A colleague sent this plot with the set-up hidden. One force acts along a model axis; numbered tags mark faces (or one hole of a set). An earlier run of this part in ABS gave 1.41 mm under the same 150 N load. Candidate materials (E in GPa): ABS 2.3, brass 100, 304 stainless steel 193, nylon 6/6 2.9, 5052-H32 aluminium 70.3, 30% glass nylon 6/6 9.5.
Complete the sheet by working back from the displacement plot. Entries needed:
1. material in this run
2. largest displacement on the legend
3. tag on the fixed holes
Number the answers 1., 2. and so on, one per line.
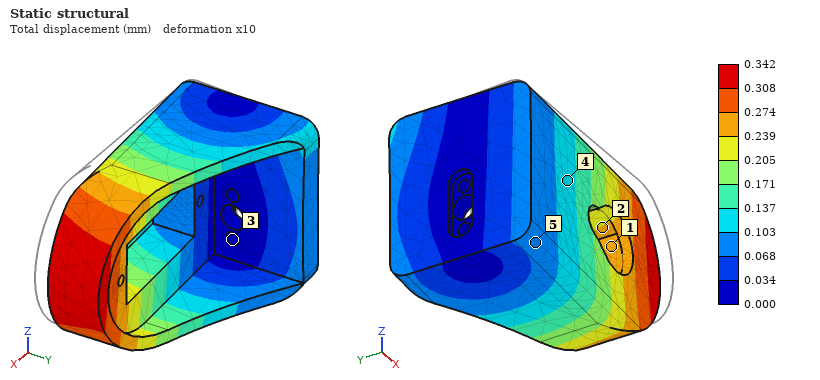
1. 30% glass nylon 6/6
2. 0.342 mm
3. 3
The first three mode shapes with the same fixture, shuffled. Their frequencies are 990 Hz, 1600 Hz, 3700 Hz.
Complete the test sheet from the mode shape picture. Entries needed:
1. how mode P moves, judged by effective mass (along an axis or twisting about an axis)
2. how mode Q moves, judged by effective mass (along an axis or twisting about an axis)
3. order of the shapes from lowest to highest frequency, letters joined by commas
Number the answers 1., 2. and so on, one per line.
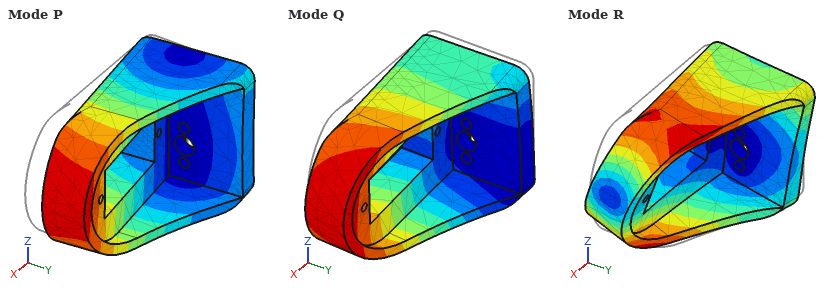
1. along Y
2. along Z
3. P, Q, R
